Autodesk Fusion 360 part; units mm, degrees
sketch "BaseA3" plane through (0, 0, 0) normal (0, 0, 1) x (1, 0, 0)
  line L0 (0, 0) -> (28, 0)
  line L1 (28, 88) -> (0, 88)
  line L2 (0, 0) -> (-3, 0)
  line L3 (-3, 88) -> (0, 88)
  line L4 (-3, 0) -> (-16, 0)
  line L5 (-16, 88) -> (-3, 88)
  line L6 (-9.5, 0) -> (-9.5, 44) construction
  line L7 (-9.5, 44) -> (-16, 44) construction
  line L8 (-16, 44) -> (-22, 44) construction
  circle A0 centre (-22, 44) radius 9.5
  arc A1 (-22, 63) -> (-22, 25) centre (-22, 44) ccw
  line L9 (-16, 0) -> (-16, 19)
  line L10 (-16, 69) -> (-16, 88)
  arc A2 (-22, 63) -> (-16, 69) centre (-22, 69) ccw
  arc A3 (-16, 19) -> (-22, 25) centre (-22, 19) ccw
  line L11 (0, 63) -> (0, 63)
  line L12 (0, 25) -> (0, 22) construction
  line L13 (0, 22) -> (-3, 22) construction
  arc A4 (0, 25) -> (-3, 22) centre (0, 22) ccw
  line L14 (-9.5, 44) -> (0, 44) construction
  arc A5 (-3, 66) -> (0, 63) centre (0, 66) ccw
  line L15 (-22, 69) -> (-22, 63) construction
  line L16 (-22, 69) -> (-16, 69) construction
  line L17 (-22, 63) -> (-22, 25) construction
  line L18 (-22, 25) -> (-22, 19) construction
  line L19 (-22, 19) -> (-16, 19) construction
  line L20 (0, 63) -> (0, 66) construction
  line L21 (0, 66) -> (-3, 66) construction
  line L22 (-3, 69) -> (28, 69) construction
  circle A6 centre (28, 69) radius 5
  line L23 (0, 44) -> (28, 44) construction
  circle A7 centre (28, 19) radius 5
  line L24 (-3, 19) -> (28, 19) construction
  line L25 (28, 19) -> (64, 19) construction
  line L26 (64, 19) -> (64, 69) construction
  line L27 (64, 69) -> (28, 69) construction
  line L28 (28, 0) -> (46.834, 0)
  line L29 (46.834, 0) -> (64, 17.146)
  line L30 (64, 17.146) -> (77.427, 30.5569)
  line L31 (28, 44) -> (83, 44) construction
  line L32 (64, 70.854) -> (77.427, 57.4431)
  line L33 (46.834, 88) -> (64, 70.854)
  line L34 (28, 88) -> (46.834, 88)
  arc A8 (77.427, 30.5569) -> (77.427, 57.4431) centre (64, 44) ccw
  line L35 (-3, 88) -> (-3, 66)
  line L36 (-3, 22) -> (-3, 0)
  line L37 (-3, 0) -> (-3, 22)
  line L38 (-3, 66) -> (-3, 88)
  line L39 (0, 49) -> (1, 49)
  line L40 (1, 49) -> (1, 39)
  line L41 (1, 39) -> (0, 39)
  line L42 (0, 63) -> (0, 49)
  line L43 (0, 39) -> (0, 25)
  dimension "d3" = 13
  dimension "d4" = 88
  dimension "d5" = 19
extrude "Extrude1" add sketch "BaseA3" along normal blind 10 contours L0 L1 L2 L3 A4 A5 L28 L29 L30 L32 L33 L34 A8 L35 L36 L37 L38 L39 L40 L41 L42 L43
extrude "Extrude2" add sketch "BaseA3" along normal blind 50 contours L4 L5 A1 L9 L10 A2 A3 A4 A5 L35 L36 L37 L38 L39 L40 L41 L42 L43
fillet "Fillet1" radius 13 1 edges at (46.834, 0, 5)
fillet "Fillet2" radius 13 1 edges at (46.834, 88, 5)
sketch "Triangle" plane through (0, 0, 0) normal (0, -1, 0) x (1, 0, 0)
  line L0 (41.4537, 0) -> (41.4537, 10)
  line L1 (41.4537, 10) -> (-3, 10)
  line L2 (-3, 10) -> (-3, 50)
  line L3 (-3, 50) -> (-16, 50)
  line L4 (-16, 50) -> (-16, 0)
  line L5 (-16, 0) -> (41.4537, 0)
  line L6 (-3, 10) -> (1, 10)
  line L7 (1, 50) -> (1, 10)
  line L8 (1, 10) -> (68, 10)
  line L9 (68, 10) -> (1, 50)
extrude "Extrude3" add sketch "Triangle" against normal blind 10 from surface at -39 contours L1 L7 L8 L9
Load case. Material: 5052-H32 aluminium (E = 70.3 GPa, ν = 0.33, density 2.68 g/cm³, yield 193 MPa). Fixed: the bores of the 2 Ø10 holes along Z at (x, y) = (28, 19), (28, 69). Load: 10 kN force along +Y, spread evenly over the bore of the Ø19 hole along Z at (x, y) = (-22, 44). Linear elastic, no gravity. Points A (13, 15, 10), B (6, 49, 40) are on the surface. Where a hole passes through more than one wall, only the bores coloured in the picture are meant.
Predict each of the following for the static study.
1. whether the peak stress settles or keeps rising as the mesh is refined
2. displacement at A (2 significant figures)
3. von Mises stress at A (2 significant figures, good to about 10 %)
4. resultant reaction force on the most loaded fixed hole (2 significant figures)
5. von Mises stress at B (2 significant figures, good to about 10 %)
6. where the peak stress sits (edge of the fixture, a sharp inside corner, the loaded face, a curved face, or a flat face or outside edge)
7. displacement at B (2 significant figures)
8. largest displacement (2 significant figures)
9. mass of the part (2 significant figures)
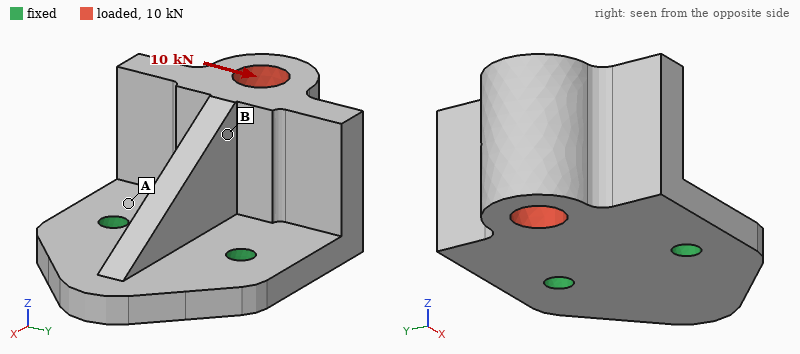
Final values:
keeps rising
0.026 mm
40 MPa
11 kN
16 MPa
edge of the fixture
0.081 mm
0.14 mm
440 g
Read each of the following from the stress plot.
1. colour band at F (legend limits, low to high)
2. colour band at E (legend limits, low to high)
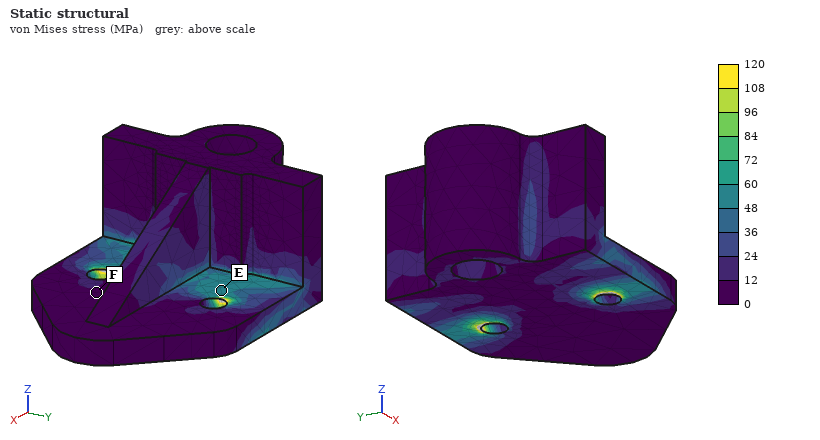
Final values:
0 to 12 MPa
48 to 60 MPa
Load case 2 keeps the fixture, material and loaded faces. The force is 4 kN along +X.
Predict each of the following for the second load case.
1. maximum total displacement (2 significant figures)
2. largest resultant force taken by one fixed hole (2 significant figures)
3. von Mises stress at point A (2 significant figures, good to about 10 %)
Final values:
0.11 mm
2.0 kN
20 MPa
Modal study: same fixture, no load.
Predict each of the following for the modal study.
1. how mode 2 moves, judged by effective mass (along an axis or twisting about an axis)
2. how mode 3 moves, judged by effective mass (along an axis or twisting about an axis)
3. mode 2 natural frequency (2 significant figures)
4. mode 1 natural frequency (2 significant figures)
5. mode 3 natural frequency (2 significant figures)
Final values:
along Y
along Z
2900 Hz
1600 Hz
5400 Hz
